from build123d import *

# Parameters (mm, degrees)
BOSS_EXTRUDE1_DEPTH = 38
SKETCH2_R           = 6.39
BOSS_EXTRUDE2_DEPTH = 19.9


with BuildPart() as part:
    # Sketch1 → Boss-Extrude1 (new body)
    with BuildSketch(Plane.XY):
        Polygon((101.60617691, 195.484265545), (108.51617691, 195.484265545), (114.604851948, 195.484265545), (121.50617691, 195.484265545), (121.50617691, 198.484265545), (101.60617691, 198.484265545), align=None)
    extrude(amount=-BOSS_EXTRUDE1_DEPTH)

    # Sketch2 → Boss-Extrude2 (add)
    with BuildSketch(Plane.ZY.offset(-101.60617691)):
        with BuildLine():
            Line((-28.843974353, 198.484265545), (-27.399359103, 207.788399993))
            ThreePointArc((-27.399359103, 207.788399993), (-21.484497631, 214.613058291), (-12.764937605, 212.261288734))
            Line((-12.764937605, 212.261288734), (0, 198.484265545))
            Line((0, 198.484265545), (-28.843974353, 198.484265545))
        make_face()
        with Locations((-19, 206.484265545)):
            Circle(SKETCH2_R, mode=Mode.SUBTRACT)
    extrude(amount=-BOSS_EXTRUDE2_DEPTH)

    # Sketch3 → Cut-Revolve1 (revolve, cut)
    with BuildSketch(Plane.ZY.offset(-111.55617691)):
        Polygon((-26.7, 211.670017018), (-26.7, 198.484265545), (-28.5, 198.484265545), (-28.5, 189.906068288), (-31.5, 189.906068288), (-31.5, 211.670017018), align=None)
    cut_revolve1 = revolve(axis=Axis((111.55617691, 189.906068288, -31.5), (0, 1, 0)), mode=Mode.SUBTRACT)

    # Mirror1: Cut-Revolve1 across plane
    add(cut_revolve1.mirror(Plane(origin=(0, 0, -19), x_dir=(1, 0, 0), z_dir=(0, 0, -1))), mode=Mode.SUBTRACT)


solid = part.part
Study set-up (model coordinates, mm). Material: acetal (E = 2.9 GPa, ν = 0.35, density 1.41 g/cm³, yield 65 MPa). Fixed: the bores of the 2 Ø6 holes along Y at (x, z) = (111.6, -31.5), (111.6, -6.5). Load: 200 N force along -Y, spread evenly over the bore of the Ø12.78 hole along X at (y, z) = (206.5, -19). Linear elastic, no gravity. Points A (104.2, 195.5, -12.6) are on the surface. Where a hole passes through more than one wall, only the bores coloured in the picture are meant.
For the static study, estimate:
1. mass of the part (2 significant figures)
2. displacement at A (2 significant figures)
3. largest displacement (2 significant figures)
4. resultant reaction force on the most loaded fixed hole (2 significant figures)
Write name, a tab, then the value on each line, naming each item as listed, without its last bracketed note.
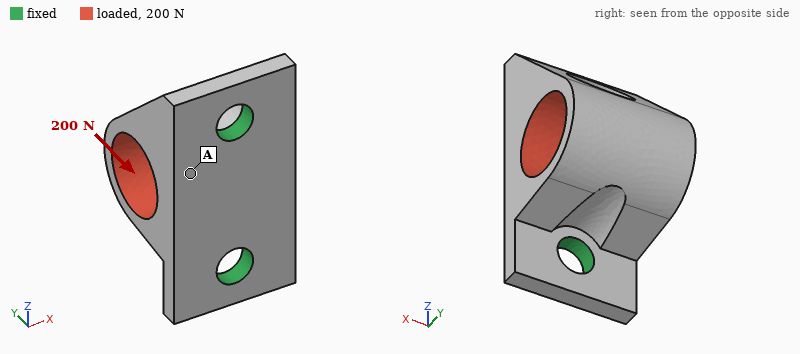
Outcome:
mass of the part	7.4 g
displacement at A	14 µm
largest displacement	25 µm
resultant reaction force on the most loaded fixed hole	110 N
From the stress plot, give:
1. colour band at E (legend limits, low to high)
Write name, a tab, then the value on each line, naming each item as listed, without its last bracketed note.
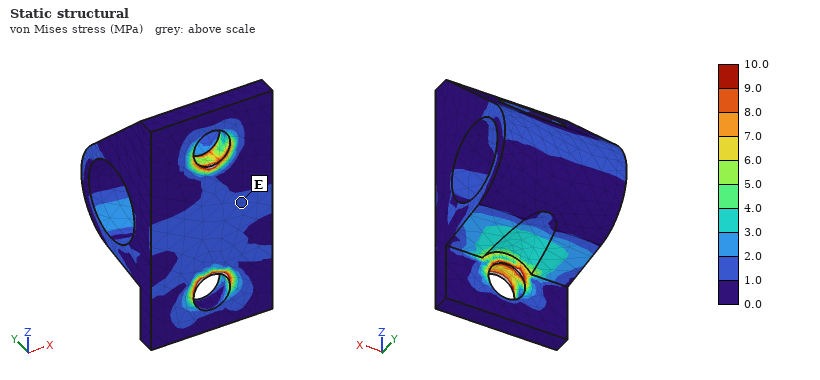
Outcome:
colour band at E	1.0 to 2.0 MPa
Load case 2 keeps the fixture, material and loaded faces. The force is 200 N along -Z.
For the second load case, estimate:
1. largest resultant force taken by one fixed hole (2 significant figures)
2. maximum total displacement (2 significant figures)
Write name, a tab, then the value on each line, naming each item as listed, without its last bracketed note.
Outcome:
largest resultant force taken by one fixed hole	130 N
maximum total displacement	61 µm
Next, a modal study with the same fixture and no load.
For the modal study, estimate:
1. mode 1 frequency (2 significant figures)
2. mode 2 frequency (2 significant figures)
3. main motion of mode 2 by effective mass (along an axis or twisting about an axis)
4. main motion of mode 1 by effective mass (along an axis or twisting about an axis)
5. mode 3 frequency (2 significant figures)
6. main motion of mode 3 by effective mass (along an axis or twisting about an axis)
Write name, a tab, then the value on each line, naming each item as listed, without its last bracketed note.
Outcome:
mode 1 frequency	3100 Hz
mode 2 frequency	5700 Hz
main motion of mode 2 by effective mass	along Z
main motion of mode 1 by effective mass	along X
mode 3 frequency	7500 Hz
main motion of mode 3 by effective mass	along Y
